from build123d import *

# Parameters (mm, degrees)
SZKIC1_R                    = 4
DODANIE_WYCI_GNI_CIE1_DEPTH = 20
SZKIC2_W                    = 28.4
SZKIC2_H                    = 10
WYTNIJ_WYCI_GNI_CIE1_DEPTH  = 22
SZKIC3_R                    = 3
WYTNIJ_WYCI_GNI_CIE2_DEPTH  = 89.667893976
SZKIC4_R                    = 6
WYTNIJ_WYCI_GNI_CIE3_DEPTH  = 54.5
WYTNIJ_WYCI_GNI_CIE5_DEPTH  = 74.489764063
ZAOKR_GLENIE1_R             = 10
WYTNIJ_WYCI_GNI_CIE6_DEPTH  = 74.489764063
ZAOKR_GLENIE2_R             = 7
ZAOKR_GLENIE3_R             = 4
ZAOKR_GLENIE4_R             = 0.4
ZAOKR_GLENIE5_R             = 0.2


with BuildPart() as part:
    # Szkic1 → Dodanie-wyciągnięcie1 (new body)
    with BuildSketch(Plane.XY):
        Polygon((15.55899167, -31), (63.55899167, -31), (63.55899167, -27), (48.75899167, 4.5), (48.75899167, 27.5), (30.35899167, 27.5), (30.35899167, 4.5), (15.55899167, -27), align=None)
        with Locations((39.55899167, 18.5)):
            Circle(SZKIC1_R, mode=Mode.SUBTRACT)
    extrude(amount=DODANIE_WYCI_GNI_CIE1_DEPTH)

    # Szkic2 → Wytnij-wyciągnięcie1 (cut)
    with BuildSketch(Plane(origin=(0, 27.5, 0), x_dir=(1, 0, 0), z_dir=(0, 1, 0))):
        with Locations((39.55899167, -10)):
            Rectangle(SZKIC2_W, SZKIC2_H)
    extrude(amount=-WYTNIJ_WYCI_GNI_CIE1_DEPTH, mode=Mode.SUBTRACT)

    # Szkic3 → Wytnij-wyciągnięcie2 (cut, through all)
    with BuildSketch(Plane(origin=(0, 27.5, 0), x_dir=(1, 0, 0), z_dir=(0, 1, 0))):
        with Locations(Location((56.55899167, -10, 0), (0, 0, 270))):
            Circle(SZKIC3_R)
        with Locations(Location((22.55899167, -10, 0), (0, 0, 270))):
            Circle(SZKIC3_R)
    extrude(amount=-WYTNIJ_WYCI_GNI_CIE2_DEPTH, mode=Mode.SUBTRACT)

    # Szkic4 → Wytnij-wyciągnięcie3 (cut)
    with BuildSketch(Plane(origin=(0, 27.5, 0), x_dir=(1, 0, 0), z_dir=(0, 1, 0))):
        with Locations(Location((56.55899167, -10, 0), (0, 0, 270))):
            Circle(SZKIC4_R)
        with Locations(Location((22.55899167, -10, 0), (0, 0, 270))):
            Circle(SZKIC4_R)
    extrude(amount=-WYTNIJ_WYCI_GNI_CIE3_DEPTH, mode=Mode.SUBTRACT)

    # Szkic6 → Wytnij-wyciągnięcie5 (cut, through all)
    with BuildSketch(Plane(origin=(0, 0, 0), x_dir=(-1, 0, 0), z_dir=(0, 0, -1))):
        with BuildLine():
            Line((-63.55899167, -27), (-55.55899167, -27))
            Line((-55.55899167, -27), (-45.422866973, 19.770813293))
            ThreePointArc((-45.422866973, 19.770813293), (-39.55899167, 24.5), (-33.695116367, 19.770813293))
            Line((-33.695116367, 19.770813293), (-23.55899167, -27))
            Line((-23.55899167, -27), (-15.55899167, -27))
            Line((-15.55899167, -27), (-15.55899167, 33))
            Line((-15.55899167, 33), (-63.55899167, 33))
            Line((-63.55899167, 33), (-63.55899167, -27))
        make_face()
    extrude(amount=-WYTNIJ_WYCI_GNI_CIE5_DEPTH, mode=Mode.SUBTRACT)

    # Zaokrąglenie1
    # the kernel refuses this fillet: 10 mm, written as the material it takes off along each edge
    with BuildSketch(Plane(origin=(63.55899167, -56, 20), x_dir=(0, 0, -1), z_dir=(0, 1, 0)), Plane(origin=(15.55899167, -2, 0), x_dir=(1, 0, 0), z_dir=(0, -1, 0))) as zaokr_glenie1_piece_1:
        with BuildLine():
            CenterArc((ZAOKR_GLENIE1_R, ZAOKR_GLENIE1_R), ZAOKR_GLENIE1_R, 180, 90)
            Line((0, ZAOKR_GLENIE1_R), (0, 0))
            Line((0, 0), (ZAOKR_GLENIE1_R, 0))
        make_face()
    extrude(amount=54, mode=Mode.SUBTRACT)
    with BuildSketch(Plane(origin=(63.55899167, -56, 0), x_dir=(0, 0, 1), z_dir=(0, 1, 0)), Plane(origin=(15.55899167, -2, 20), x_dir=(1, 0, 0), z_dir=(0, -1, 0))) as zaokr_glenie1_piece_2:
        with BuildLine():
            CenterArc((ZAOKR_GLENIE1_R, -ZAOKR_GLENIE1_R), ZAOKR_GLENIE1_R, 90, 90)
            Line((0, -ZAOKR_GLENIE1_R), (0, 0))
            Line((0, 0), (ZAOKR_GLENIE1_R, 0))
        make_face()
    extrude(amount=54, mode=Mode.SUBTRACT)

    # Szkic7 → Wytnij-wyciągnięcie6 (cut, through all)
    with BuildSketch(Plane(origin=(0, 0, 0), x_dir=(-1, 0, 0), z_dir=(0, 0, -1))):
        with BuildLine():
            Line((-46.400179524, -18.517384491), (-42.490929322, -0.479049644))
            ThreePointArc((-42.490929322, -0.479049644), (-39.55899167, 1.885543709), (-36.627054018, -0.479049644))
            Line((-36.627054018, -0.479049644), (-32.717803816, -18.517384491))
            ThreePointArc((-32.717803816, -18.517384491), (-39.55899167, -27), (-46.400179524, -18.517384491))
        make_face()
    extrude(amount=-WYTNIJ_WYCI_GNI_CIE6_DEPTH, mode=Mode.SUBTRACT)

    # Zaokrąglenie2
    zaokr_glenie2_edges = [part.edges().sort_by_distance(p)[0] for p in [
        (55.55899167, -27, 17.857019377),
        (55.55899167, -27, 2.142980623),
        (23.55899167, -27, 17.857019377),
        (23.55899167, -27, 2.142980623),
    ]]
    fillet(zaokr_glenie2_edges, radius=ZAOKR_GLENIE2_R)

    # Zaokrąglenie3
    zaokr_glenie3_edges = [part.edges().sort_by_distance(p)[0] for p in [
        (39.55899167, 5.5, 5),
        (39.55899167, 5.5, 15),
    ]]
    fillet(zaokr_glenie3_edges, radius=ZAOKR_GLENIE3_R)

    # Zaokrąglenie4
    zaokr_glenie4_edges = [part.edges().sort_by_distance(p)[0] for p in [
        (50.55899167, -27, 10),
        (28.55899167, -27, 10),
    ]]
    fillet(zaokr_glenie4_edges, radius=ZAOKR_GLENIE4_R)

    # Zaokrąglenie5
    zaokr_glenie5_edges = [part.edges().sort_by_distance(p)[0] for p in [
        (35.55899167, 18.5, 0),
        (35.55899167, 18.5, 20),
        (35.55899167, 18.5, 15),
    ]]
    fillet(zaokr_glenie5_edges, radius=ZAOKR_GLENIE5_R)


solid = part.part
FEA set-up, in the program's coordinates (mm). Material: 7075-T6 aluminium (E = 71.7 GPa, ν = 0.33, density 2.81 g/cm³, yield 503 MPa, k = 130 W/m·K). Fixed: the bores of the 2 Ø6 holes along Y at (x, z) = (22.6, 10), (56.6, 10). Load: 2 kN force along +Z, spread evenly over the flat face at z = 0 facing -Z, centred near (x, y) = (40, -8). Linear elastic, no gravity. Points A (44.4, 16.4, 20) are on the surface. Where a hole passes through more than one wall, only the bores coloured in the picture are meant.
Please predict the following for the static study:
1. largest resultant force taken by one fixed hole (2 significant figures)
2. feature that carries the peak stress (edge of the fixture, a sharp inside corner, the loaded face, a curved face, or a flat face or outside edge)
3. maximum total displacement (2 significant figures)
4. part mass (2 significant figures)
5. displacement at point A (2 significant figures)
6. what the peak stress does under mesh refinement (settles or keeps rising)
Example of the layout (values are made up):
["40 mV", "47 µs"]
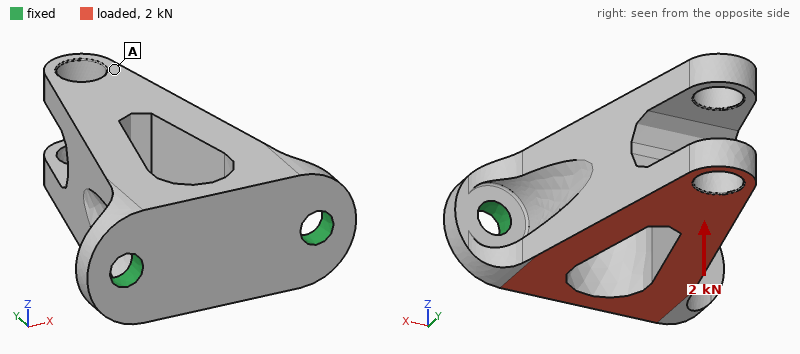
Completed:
["1.0 kN", "edge of the fixture", "0.31 mm", "43 g", "0.24 mm", "keeps rising"]
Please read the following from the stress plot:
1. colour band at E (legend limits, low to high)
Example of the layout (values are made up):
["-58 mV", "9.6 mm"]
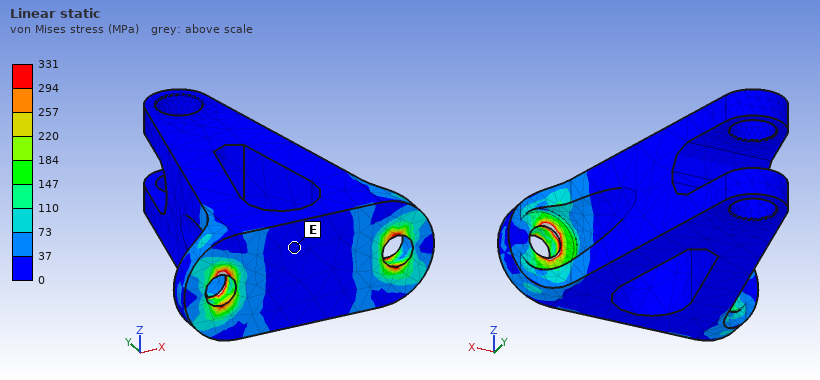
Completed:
["0 to 37 MPa"]
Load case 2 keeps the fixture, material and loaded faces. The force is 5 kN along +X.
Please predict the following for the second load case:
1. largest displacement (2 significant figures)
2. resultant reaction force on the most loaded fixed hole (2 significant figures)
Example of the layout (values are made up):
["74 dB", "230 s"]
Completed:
["0.16 mm", "4.5 kN"]
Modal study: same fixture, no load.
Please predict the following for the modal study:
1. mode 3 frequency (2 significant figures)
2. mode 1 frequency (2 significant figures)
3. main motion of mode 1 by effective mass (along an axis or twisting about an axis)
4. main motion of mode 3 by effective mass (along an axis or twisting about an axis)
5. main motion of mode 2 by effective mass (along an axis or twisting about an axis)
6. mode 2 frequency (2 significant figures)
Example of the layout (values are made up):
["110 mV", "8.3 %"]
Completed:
["11 kHz", "3000 Hz", "along Z", "twisting about Y", "along X", "6600 Hz"]
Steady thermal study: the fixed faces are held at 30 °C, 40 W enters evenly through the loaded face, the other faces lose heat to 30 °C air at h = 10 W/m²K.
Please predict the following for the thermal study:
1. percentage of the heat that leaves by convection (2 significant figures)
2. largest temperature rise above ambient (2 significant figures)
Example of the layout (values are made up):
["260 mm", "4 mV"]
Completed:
["3.1 %", "42 K"]
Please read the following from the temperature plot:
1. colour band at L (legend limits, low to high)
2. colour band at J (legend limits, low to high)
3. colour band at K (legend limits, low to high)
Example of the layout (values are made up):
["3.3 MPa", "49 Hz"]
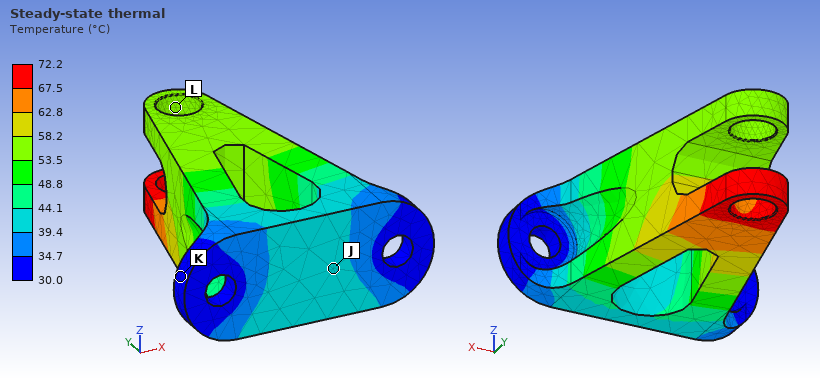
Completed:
["53.5 to 58.2 °C", "39.4 to 44.1 °C", "30.0 to 34.7 °C"]
